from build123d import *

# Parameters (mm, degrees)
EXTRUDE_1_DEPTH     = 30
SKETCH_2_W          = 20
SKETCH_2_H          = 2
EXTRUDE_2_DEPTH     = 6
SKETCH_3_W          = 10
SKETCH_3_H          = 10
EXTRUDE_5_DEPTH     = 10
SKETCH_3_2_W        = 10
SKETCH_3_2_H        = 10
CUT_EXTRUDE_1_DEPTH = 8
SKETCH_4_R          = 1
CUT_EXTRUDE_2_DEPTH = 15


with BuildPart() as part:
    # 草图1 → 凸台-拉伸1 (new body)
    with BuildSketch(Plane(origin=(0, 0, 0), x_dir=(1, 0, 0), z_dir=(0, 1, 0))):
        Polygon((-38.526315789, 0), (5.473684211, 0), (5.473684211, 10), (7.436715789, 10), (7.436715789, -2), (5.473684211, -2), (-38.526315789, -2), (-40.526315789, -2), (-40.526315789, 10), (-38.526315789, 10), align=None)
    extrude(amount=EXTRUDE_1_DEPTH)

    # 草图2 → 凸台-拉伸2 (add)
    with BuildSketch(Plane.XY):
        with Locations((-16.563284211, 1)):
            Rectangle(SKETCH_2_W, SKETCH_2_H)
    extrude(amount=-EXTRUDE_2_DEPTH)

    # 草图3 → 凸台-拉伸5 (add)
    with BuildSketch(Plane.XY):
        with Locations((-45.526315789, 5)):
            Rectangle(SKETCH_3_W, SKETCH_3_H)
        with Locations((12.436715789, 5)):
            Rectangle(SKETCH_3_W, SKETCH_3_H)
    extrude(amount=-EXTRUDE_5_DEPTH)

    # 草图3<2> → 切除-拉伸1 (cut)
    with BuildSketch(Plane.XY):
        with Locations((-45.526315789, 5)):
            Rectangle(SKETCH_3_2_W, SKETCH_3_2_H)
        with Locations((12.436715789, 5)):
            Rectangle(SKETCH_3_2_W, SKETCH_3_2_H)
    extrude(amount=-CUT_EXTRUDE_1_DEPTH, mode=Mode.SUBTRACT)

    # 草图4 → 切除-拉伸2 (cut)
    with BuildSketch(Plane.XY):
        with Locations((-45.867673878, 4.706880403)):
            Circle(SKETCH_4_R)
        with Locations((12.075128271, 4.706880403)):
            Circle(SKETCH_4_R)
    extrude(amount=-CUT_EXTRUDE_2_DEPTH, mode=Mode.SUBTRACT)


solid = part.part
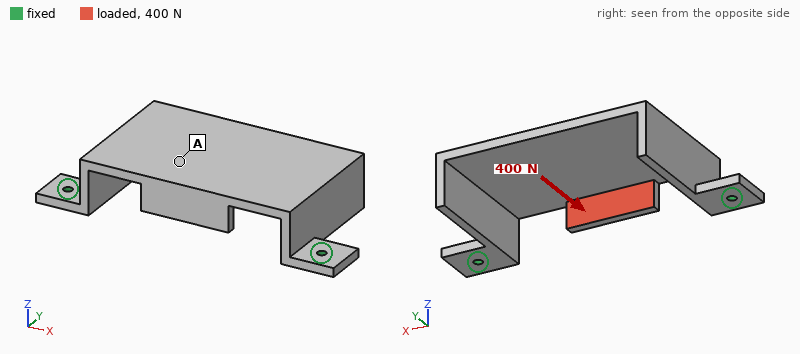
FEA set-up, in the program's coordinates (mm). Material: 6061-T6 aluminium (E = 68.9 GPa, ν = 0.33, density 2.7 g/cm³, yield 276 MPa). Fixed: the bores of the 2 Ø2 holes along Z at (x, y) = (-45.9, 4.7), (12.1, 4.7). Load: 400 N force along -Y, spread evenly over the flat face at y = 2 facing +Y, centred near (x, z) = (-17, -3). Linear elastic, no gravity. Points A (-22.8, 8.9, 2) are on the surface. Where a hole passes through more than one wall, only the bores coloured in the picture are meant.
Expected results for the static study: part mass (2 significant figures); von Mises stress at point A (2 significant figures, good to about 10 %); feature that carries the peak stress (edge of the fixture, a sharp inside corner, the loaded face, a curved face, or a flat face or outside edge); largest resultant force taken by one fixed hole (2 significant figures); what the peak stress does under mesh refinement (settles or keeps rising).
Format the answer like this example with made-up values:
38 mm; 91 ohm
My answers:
13 g; 31 MPa; edge of the fixture; 200 N; keeps rising
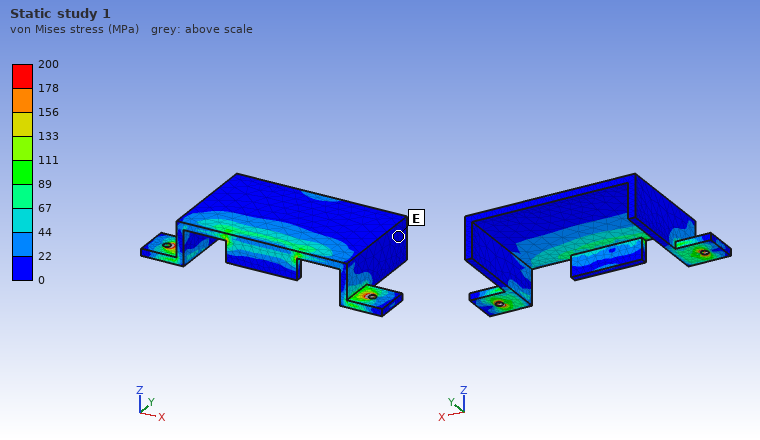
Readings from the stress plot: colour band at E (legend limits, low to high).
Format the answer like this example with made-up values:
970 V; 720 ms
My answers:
0 to 22 MPa
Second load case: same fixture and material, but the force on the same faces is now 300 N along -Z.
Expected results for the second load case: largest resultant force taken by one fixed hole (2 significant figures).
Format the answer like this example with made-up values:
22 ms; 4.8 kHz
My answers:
220 N
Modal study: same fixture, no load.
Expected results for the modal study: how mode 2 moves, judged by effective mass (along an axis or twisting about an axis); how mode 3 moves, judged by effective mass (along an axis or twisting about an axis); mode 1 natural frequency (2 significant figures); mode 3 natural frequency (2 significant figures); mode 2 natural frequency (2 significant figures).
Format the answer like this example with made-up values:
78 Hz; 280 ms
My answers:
along X; along X; 1500 Hz; 3600 Hz; 2600 Hz
